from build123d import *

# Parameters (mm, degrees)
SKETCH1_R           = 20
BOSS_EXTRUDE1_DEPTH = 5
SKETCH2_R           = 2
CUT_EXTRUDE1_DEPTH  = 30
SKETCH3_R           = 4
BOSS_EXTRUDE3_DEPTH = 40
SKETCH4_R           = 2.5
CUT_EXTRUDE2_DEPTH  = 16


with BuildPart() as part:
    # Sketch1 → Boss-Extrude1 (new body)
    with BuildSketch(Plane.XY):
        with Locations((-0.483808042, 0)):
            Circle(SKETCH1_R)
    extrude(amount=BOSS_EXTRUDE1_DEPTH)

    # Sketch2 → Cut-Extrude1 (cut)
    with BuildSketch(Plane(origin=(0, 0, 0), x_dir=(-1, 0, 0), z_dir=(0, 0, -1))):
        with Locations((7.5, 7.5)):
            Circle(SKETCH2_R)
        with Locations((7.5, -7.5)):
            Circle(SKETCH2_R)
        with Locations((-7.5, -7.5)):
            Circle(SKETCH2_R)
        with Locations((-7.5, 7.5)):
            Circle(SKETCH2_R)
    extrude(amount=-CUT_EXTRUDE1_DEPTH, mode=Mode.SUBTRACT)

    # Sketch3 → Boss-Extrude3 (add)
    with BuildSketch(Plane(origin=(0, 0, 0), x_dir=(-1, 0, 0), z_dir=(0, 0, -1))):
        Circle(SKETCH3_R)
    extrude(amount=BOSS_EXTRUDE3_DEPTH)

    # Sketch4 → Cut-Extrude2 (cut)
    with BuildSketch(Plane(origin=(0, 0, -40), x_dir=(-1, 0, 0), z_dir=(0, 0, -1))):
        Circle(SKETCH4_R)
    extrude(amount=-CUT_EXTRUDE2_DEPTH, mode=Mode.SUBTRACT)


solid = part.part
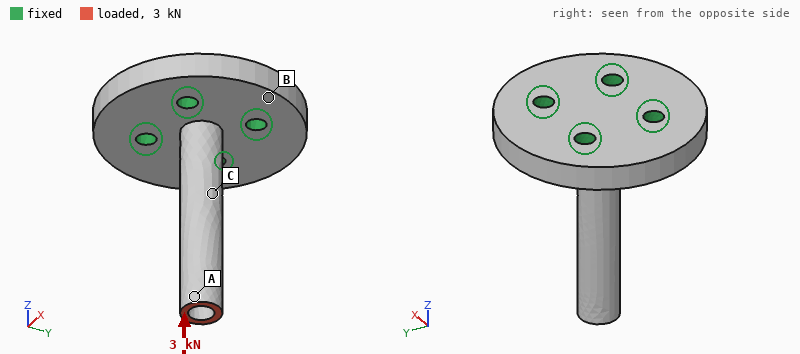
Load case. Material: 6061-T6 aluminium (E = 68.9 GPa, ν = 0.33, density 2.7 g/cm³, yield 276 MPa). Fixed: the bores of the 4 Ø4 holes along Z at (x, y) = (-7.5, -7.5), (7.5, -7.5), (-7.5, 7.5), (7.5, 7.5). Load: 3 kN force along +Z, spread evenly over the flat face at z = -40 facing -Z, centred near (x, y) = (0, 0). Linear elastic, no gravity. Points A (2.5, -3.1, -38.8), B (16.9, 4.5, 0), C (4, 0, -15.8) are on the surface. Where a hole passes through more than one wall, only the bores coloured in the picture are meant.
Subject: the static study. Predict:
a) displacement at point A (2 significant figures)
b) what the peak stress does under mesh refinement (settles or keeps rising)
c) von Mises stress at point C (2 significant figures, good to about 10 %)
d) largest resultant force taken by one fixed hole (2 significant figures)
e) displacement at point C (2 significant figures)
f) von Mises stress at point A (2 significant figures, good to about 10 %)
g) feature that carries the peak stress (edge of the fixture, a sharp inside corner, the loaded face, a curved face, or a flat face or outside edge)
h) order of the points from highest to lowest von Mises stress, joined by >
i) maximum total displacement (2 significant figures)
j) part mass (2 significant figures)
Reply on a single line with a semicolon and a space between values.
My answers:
51 µm; keeps rising; 60 MPa; 770 N; 22 µm; 98 MPa; edge of the fixture; A > C > B; 53 µm; 21 g
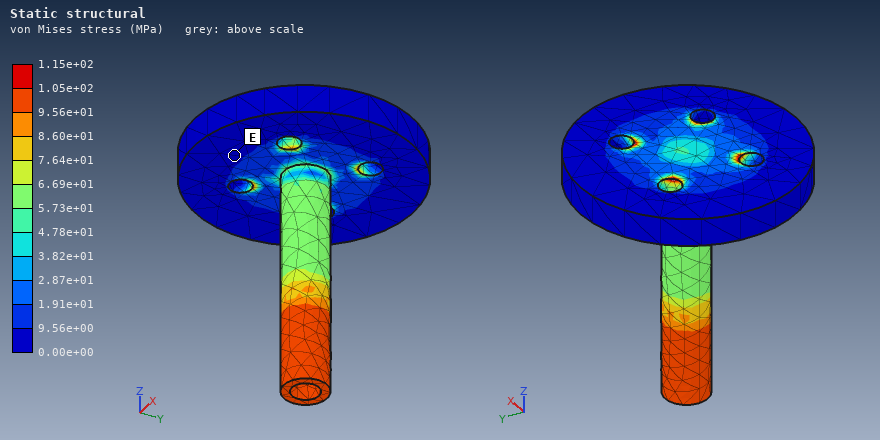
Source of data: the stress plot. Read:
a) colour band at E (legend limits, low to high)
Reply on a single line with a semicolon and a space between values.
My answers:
0.00e+00 to 9.56e+00 MPa
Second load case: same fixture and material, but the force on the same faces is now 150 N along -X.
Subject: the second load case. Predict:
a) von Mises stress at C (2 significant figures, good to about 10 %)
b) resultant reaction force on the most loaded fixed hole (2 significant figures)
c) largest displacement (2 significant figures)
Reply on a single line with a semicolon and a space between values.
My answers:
74 MPa; 250 N; 0.29 mm
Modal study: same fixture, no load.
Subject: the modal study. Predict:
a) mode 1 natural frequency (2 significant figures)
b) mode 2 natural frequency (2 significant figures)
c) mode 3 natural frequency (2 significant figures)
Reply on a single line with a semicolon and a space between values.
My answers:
3800 Hz; 3800 Hz; 19 kHz
